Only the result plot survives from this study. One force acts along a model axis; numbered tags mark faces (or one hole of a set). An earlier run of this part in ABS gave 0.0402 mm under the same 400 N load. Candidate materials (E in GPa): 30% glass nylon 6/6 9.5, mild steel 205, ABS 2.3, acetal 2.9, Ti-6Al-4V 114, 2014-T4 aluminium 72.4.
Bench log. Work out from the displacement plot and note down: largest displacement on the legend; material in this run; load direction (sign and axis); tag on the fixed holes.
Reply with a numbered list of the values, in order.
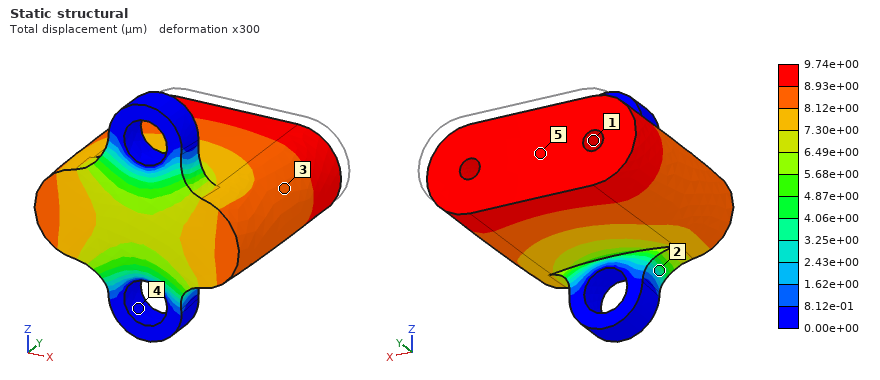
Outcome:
1. 9.74e+00 µm
2. 30% glass nylon 6/6
3. -Y
4. 4
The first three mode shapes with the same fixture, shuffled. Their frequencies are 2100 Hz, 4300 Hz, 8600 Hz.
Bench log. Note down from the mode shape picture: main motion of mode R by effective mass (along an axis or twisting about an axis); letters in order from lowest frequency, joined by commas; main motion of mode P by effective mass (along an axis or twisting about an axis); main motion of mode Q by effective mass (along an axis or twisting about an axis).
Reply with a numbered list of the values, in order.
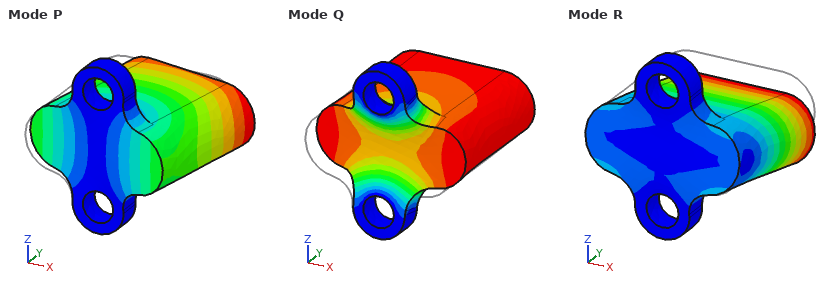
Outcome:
1. along Z
2. P, R, Q
3. along X
4. along Y
